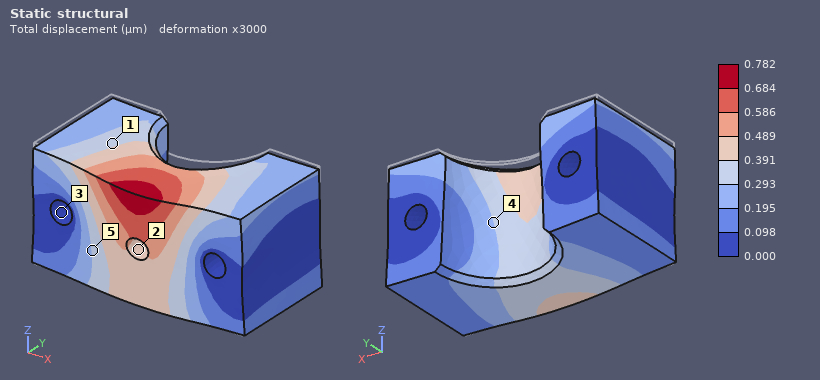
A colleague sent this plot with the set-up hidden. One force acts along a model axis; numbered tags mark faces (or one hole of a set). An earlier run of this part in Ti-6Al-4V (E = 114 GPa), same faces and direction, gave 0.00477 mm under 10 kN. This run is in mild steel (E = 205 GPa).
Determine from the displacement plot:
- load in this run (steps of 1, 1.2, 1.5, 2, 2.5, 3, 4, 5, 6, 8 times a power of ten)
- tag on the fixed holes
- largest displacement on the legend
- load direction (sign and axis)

3 kN
3
0.782 µm
-Z
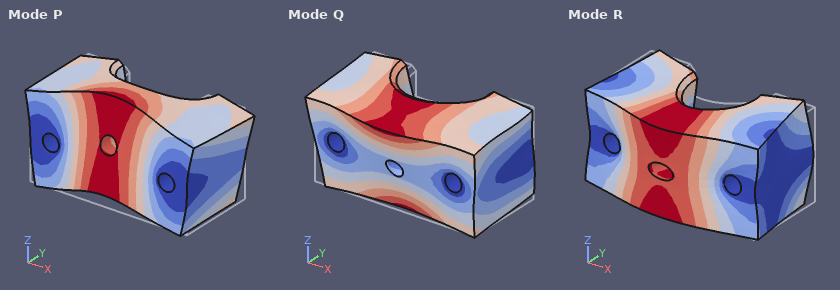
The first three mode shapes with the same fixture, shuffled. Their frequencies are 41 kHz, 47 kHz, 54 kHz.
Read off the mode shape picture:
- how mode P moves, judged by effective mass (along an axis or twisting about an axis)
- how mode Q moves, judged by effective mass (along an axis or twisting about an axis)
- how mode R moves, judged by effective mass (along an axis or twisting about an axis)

along Z
twisting about X
along Y
